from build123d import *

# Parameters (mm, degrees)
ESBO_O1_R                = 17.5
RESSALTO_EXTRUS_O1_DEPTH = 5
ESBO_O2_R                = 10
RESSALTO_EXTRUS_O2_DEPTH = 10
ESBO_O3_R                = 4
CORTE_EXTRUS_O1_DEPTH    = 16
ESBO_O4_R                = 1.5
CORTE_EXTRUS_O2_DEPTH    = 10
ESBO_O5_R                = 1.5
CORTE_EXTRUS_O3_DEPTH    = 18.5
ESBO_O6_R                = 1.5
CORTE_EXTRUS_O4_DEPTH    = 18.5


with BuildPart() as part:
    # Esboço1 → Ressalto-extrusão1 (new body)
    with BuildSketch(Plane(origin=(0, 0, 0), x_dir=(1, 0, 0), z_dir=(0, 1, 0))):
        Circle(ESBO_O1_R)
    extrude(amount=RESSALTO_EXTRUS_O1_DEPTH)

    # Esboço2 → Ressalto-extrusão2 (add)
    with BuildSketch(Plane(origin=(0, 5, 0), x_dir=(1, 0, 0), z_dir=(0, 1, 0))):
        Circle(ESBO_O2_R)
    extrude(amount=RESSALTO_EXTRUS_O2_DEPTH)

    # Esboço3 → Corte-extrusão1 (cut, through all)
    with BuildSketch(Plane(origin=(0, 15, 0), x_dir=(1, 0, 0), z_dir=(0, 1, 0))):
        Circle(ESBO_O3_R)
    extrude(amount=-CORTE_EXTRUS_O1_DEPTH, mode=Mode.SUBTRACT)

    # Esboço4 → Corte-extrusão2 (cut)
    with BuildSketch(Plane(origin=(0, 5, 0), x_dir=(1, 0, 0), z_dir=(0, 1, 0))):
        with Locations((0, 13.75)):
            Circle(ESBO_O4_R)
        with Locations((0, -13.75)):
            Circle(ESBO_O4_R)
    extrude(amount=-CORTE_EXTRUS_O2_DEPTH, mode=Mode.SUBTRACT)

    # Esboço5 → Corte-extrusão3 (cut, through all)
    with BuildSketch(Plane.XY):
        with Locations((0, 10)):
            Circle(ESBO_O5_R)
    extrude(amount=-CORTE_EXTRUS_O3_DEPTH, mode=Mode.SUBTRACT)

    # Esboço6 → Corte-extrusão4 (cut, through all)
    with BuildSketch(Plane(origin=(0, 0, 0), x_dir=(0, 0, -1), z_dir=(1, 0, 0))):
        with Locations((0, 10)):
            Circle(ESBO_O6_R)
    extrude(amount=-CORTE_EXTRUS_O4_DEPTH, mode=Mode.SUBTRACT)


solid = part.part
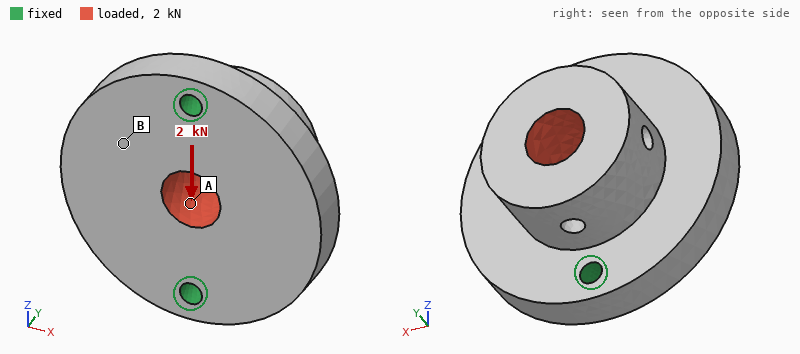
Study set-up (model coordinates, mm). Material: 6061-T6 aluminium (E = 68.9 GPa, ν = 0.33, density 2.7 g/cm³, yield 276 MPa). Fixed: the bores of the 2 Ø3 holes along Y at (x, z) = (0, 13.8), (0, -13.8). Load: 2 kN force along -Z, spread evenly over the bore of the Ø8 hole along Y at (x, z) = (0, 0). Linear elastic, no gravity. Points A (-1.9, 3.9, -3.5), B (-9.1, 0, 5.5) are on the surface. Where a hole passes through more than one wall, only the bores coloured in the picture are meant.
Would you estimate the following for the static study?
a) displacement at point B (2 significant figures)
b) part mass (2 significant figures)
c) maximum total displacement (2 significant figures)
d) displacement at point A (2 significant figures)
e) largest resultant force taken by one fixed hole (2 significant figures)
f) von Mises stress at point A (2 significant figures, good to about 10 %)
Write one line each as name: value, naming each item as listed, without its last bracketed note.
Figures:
displacement at point B: 1.9 µm
part mass: 19 g
maximum total displacement: 6.6 µm
displacement at point A: 2.5 µm
largest resultant force taken by one fixed hole: 1.1 kN
von Mises stress at point A: 11 MPa
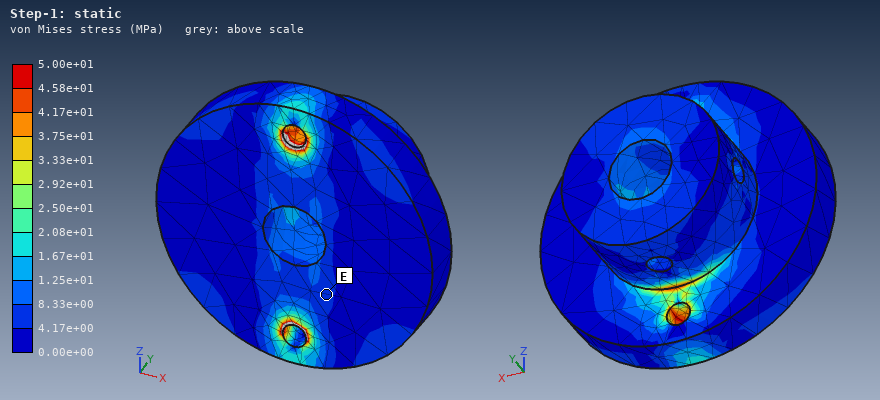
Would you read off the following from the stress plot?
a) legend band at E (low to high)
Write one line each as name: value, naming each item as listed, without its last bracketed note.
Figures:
legend band at E: 4.17e+00 to 8.33e+00 MPa
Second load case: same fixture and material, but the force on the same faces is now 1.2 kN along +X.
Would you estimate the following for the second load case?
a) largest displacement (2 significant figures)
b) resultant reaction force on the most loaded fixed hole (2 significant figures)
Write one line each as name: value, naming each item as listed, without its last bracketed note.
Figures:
largest displacement: 21 µm
resultant reaction force on the most loaded fixed hole: 600 N
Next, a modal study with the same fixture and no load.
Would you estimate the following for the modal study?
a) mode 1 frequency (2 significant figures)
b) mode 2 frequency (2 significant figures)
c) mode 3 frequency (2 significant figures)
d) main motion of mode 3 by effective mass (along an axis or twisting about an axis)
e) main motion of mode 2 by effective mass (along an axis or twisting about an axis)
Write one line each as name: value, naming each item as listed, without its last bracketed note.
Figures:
mode 1 frequency: 9000 Hz
mode 2 frequency: 18 kHz
mode 3 frequency: 28 kHz
main motion of mode 3 by effective mass: along Z
main motion of mode 2 by effective mass: along Y
